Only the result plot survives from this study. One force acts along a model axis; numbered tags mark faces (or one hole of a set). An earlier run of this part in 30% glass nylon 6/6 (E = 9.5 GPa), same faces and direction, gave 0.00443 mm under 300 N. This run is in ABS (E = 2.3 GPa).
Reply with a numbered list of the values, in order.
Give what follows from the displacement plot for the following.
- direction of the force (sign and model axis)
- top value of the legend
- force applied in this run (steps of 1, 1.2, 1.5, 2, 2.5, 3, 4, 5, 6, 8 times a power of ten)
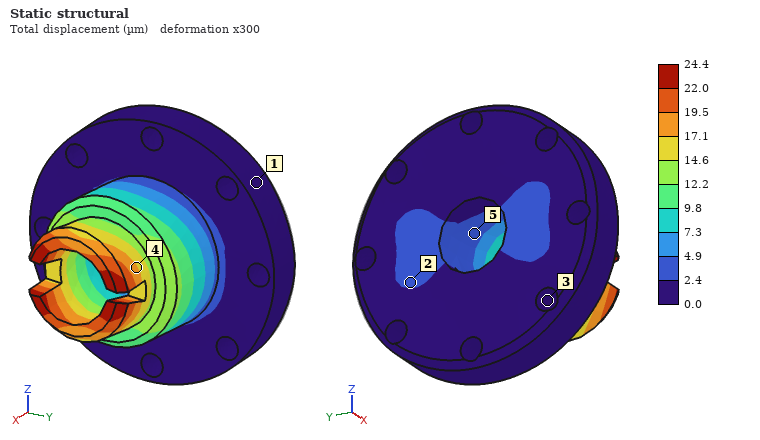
1. -Y
2. 24.4 µm
3. 400 N
